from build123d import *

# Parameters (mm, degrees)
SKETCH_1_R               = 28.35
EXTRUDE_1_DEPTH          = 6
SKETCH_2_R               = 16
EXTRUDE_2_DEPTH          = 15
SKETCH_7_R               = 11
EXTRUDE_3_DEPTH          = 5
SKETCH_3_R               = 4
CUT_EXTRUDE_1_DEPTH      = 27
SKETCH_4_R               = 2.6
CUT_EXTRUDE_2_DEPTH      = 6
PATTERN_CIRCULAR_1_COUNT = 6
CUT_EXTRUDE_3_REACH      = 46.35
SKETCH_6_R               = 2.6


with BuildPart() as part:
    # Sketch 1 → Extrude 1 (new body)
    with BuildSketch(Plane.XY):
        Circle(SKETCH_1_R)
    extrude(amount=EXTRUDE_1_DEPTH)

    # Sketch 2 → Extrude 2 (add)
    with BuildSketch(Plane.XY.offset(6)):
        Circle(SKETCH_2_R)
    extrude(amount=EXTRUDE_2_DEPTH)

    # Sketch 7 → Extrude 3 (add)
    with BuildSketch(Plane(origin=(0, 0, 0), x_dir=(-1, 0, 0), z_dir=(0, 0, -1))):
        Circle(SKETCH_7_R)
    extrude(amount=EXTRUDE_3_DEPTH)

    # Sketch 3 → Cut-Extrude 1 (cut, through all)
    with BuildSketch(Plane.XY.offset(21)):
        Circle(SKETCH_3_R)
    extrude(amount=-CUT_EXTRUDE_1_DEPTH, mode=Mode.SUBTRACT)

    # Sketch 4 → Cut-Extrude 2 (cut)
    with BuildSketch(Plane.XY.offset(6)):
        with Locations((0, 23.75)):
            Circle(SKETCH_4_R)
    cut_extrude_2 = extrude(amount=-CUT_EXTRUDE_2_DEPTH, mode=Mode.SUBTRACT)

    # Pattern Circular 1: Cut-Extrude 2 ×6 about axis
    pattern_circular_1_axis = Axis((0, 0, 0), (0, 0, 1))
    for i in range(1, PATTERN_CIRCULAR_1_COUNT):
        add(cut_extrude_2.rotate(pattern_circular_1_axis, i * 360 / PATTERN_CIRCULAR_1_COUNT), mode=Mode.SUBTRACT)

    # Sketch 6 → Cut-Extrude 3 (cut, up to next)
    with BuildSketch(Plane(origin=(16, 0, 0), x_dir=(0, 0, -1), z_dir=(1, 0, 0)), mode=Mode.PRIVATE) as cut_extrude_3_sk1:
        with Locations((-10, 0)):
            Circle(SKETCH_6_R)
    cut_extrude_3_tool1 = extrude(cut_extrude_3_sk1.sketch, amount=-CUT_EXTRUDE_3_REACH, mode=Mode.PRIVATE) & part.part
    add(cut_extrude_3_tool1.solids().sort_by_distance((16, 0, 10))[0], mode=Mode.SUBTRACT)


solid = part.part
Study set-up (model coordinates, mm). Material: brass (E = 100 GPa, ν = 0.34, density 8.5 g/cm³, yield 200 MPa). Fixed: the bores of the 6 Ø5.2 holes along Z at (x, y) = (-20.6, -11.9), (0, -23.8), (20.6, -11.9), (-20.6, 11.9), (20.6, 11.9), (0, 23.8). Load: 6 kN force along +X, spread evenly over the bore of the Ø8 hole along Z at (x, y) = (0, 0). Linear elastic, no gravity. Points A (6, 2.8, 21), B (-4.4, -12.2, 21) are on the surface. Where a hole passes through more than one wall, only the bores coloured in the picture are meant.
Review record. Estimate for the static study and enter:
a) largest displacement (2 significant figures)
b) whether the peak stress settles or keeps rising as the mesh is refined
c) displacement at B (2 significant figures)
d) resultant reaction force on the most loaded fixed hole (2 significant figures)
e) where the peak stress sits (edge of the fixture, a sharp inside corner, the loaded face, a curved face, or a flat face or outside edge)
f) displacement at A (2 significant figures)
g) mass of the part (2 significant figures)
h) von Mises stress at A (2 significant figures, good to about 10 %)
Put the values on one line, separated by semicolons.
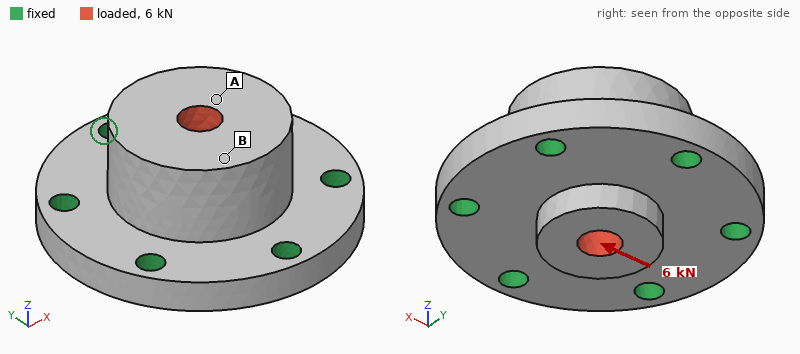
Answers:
6.0 µm; keeps rising; 4.8 µm; 1.4 kN; edge of the fixture; 5.6 µm; 230 g; 9.0 MPa
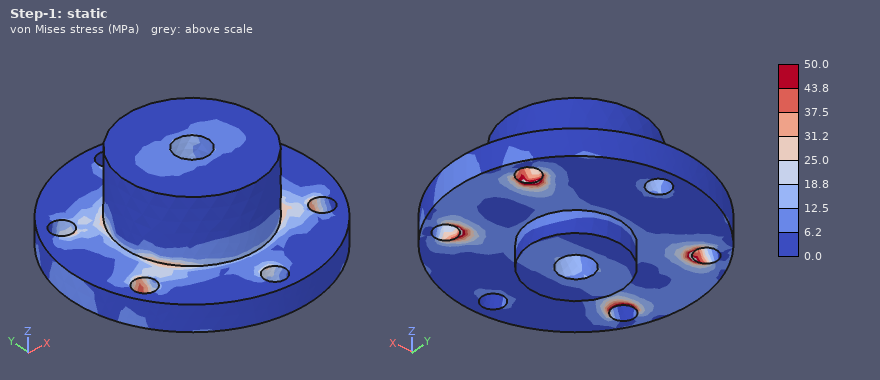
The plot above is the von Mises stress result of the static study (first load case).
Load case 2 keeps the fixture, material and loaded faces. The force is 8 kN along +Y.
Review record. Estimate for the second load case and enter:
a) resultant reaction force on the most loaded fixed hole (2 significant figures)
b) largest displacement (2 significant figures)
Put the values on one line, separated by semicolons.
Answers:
2.1 kN; 8.0 µm
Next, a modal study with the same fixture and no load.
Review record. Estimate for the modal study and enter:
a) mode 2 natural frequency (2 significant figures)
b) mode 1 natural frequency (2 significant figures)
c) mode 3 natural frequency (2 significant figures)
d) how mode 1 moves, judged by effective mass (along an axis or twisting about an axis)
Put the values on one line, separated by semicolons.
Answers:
14 kHz; 13 kHz; 14 kHz; along Z
